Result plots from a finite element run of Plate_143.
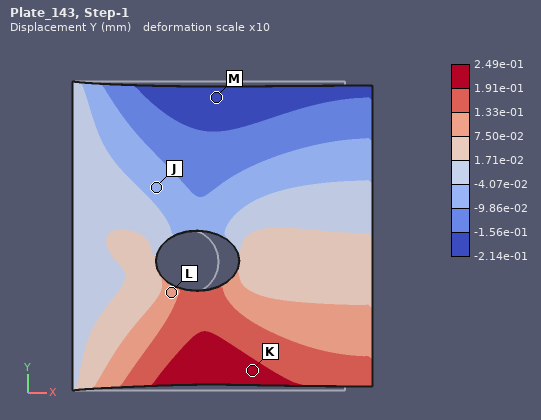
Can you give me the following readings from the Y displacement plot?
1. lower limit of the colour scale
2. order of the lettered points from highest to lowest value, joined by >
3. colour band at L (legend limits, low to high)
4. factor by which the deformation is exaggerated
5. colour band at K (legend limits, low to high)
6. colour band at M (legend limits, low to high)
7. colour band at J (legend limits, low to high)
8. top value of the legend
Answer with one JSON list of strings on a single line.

["-2.14e-01 mm", "K > L > J > M", "7.50e-02 to 1.33e-01 mm", "10", "1.91e-01 to 2.49e-01 mm", "-2.14e-01 to -1.56e-01 mm", "-9.86e-02 to -4.07e-02 mm", "2.49e-01 mm"]
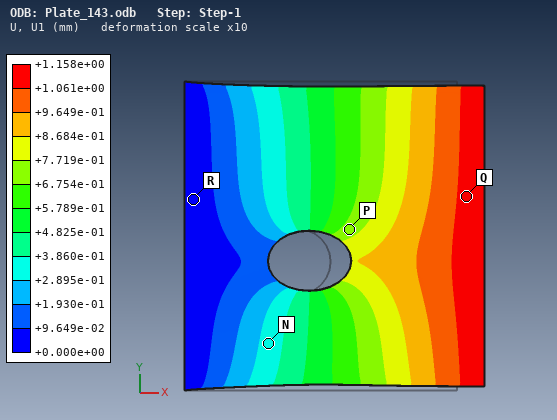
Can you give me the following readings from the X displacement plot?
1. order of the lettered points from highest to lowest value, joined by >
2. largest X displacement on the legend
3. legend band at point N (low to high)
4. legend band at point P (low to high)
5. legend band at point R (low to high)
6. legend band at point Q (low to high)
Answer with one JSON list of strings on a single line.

["Q > P > N > R", "+1.158e+00 mm", "+2.895e-01 to +3.860e-01 mm", "+6.754e-01 to +7.719e-01 mm", "+0.000e+00 to +9.649e-02 mm", "+1.061e+00 to +1.158e+00 mm"]
